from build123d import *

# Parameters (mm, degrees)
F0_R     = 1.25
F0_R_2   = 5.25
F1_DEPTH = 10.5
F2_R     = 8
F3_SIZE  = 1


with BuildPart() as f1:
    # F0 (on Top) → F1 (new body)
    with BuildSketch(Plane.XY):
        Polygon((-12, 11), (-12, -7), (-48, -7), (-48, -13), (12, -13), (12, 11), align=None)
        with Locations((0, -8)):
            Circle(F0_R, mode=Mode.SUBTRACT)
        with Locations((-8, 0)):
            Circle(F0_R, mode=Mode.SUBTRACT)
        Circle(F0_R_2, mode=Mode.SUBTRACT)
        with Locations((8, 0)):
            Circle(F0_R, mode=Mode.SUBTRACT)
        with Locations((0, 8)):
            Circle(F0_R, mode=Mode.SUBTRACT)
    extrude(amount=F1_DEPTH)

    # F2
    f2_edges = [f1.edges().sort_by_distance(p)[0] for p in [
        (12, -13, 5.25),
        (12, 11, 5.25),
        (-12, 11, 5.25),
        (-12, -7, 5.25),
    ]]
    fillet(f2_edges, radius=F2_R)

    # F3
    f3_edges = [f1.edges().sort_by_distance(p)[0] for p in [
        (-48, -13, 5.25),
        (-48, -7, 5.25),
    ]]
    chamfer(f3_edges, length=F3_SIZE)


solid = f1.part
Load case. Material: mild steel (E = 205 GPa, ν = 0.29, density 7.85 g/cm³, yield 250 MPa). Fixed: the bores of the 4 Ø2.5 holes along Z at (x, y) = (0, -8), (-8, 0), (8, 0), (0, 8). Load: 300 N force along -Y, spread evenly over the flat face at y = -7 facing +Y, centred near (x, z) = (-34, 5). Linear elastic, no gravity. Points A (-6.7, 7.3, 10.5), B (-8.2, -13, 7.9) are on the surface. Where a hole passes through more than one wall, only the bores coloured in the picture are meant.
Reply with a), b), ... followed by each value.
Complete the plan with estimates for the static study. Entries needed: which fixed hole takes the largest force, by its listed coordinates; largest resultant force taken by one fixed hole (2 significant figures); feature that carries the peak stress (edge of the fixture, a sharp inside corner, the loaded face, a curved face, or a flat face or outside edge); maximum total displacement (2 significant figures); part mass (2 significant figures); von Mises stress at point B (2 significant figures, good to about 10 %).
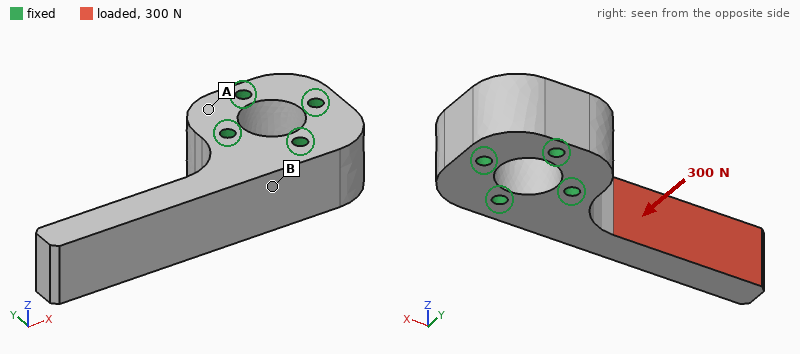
a) (-8, 0)
b) 770 N
c) a curved face
d) 51 µm
e) 54 g
f) 27 MPa
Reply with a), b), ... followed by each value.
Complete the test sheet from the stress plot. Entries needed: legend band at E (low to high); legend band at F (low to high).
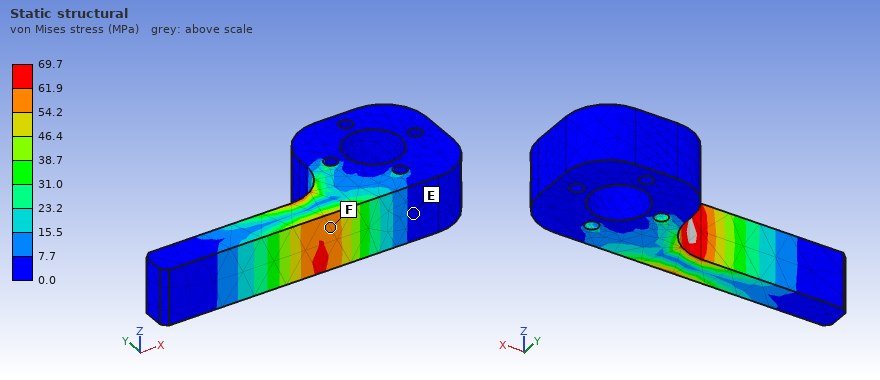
a) 0.0 to 7.7 MPa
b) 54.2 to 61.9 MPa
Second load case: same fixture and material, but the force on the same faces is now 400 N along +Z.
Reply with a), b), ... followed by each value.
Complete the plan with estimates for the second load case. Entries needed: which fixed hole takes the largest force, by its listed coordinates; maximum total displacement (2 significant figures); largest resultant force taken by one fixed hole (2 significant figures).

a) (-8, 0)
b) 43 µm
c) 640 N
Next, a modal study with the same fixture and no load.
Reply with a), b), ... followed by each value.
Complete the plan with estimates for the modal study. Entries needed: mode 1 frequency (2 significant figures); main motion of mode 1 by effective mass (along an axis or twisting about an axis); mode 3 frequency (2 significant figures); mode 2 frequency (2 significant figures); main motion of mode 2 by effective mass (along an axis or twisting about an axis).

a) 4000 Hz
b) along Y
c) 18 kHz
d) 5000 Hz
e) along Z
